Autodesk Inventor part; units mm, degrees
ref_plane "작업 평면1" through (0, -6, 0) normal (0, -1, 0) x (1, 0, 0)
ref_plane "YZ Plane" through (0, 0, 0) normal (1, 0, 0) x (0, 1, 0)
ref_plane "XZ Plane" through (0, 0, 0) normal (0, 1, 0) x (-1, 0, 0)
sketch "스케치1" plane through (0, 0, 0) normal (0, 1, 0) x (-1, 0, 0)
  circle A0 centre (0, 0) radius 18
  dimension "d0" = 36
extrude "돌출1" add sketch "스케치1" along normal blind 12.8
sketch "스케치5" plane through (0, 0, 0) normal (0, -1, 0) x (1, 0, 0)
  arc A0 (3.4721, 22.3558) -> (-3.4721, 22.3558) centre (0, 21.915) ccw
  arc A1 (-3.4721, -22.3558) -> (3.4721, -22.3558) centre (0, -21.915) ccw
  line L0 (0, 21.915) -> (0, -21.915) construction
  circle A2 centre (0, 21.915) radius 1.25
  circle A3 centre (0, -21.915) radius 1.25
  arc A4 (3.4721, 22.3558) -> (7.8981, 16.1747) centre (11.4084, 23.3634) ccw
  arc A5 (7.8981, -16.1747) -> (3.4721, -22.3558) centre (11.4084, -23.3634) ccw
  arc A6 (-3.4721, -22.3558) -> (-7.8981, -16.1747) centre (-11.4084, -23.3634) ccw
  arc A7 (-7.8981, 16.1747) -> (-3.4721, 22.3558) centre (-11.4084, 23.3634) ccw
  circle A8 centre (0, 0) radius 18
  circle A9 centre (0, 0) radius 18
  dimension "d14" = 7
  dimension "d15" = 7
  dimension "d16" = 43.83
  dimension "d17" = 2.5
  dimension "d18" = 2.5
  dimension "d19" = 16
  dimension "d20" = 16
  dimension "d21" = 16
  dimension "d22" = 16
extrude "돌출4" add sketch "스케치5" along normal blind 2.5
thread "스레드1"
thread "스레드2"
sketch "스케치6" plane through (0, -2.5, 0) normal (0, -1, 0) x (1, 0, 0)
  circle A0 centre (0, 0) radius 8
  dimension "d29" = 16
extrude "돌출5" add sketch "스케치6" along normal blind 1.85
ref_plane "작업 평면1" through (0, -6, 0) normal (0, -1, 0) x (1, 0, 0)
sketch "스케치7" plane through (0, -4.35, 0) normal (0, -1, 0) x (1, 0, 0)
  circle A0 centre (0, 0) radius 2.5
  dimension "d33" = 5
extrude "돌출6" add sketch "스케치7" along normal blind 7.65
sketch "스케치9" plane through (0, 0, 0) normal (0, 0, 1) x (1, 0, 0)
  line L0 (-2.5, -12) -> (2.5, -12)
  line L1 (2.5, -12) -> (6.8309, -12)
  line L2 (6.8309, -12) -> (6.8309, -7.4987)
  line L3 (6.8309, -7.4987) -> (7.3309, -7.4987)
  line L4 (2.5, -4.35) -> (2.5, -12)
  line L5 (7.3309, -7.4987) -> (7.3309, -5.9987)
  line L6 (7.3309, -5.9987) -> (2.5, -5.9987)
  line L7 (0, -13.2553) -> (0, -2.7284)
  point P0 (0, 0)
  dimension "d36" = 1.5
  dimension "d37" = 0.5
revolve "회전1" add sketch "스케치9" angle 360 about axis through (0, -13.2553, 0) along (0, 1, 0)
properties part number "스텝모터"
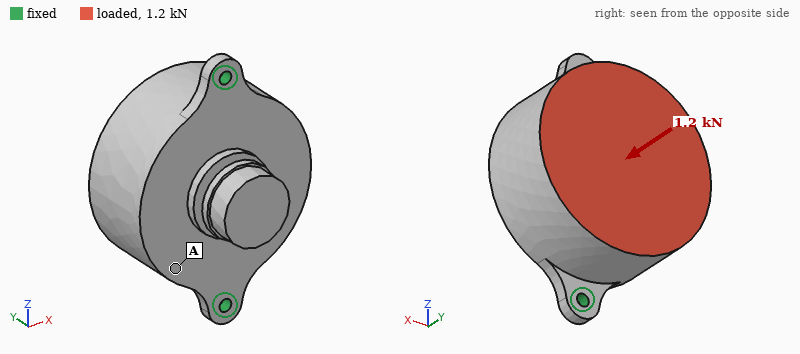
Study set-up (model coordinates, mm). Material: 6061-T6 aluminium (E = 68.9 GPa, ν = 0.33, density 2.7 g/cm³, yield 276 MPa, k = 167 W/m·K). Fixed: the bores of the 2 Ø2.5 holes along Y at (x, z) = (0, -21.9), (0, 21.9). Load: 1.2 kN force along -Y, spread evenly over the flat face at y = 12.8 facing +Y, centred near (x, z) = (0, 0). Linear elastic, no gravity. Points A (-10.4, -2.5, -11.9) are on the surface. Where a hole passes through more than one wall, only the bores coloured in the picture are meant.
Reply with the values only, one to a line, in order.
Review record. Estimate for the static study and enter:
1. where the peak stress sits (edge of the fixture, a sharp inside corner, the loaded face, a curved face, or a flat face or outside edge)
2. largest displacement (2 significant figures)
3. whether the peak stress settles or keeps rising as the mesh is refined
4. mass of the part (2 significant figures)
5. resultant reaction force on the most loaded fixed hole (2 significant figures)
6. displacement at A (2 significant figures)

edge of the fixture
17 µm
keeps rising
46 g
680 N
15 µm
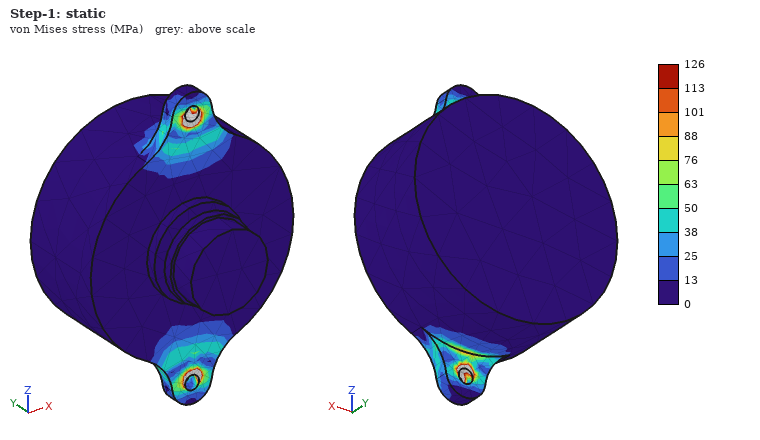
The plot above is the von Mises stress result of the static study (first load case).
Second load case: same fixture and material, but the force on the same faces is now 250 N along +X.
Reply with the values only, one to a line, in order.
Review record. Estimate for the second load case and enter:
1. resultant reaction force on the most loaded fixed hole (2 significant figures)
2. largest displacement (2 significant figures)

130 N
0.14 mm
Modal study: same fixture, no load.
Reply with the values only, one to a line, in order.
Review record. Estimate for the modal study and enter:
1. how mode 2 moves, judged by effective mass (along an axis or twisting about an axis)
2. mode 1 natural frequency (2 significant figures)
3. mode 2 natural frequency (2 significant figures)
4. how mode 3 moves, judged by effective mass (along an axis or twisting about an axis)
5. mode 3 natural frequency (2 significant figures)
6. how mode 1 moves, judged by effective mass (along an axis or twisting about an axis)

along Y
1600 Hz
6500 Hz
along X
9900 Hz
along X
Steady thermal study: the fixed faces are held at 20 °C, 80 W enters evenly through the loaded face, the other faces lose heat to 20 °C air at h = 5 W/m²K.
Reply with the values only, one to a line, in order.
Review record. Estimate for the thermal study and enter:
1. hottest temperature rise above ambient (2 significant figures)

75 K
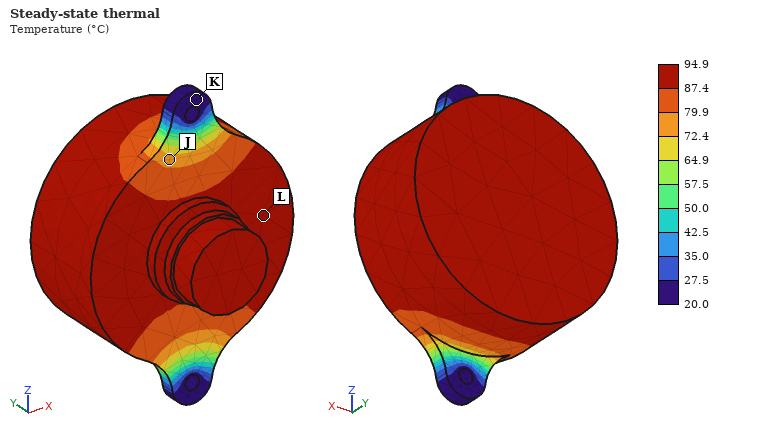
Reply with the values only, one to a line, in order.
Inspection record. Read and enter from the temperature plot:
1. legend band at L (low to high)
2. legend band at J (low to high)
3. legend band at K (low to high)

87.4 to 94.9 °C
72.4 to 79.9 °C
20.0 to 27.5 °C
